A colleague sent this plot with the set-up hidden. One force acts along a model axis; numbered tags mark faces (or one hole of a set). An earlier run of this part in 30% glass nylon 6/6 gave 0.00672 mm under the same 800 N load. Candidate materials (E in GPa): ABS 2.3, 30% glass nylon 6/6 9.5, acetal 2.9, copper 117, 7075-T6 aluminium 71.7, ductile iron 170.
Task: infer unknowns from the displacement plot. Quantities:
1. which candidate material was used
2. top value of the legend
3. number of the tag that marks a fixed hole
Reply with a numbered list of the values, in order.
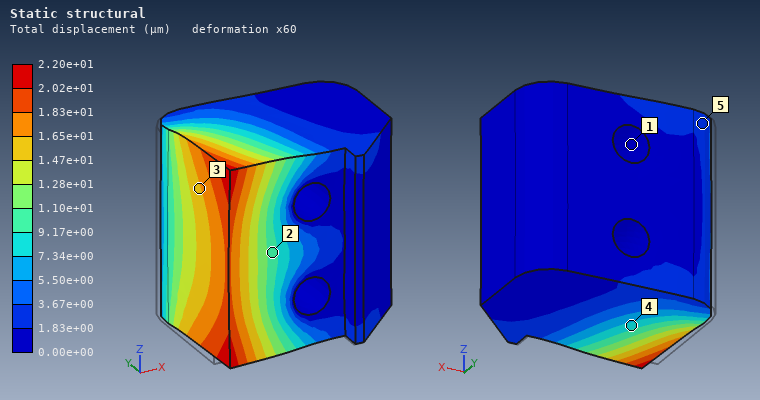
1. acetal
2. 2.20e+01 µm
3. 1
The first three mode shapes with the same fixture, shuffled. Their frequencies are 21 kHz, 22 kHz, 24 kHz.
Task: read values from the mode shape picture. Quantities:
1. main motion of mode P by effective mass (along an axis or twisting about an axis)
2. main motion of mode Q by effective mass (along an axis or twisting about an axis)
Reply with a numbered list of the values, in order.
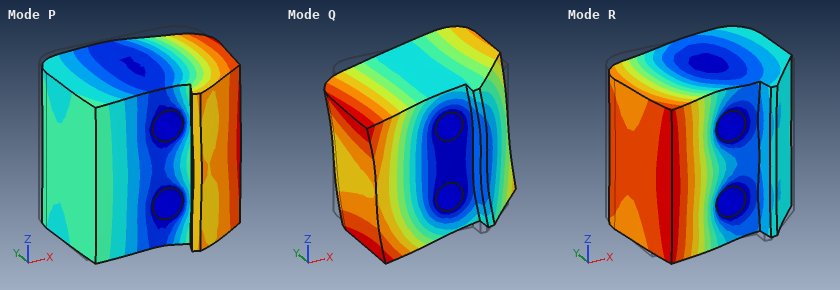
1. along Y
2. twisting about Y
